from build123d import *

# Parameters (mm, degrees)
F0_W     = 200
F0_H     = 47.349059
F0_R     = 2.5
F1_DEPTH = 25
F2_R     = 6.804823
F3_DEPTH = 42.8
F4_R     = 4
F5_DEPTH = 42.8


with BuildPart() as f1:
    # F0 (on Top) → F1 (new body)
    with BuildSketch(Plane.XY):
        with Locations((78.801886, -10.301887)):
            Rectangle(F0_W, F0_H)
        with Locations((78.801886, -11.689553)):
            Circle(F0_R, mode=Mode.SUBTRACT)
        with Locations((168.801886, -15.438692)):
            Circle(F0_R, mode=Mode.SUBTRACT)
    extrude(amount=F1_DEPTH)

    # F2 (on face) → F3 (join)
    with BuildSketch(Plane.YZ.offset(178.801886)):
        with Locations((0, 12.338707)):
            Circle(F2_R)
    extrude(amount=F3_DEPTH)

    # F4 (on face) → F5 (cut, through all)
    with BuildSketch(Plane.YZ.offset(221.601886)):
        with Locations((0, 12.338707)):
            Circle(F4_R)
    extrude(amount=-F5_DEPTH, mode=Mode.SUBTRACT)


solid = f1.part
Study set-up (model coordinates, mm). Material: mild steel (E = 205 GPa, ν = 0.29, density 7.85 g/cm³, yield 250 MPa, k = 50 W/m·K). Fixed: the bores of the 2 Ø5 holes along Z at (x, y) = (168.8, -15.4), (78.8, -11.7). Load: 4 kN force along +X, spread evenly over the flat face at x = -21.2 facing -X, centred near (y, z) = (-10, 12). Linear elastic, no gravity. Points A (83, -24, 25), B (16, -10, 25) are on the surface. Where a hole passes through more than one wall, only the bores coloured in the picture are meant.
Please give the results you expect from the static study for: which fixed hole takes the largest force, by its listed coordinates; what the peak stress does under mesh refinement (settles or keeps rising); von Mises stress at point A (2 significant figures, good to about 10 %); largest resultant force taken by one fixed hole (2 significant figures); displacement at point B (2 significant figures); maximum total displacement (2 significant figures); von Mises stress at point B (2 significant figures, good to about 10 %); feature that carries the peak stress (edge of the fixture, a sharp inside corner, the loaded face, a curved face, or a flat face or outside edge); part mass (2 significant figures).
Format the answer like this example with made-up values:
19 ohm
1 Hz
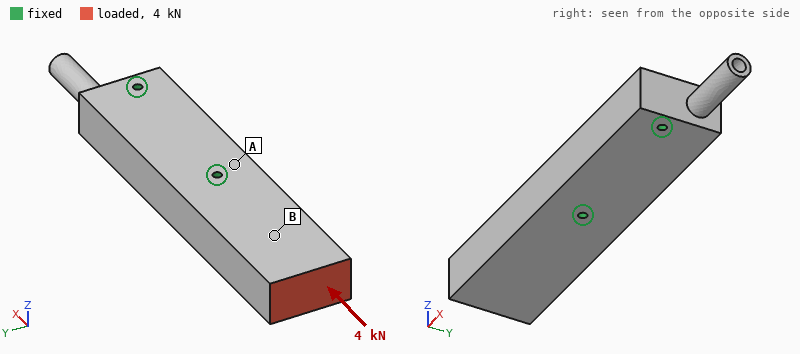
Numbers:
(78.8, -11.7)
keeps rising
1.8 MPa
3.4 kN
1.3 µm
2.0 µm
3.4 MPa
edge of the fixture
1.9 kg
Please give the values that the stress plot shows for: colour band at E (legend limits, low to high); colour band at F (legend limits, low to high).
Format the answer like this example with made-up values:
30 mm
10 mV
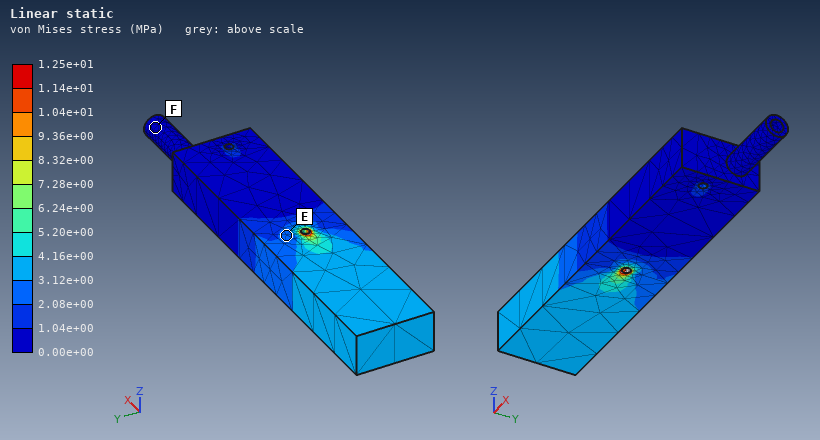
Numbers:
2.08e+00 to 3.12e+00 MPa
0.00e+00 to 1.04e+00 MPa
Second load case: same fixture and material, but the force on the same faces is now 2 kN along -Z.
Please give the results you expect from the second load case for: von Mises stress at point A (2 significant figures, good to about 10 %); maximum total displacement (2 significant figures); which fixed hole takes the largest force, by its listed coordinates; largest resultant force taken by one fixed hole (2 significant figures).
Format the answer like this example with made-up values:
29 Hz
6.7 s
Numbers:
22 MPa
69 µm
(78.8, -11.7)
2.9 kN
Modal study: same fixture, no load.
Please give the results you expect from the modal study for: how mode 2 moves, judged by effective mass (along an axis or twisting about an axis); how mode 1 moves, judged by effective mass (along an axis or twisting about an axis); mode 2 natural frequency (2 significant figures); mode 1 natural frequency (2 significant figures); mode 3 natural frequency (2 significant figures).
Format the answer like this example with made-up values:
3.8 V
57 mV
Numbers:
along Y
along Z
2300 Hz
1700 Hz
4900 Hz
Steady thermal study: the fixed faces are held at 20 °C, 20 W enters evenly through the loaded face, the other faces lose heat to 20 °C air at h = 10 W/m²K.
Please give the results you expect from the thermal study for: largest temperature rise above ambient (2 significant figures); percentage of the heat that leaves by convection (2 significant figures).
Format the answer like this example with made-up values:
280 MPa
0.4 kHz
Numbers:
33 K
13 %
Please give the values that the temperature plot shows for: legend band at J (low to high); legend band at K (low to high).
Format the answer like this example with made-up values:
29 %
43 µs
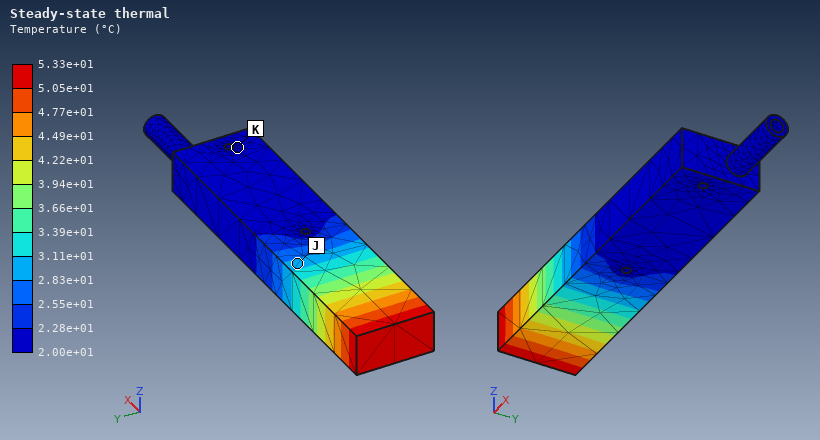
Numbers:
2.83e+01 to 3.11e+01 °C
2.00e+01 to 2.28e+01 °C
